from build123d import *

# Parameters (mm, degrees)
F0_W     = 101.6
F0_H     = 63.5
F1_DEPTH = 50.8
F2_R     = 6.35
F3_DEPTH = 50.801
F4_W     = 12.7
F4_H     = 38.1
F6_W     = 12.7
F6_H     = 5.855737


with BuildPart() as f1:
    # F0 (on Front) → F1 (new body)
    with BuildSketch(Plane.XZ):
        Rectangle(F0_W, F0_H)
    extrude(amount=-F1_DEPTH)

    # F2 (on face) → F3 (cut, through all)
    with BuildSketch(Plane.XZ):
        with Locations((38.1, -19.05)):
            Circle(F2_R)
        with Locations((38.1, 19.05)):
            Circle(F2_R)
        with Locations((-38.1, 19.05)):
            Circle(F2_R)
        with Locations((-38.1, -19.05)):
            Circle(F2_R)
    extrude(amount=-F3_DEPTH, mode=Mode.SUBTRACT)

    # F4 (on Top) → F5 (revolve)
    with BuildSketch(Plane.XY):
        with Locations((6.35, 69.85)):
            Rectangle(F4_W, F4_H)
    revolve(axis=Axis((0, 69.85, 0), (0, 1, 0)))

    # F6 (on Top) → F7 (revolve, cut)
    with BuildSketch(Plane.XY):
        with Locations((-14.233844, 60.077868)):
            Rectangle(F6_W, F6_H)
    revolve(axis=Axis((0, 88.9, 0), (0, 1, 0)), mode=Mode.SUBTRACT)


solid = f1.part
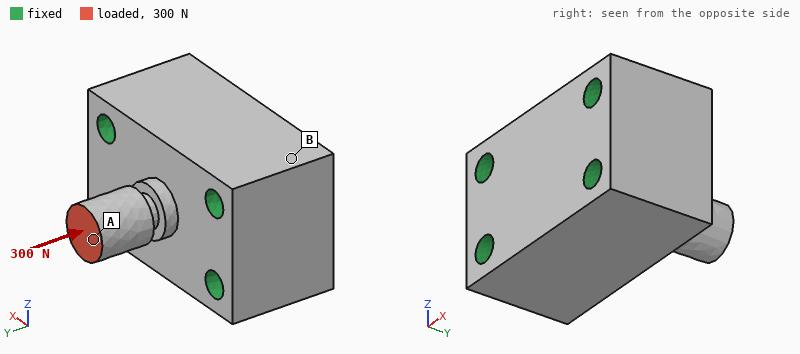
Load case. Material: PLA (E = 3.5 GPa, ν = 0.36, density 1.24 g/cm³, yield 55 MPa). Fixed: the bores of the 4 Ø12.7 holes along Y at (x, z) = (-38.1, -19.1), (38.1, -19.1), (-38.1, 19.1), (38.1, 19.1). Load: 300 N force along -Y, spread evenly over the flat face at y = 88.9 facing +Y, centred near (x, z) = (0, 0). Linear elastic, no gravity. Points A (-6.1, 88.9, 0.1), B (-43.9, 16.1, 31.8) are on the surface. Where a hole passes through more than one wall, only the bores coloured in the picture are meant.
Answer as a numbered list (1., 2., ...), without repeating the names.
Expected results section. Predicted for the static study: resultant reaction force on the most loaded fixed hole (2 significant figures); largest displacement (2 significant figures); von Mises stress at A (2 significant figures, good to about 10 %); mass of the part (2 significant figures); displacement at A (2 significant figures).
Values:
1. 80 N
2. 13 µm
3. 0.59 MPa
4. 400 g
5. 13 µm
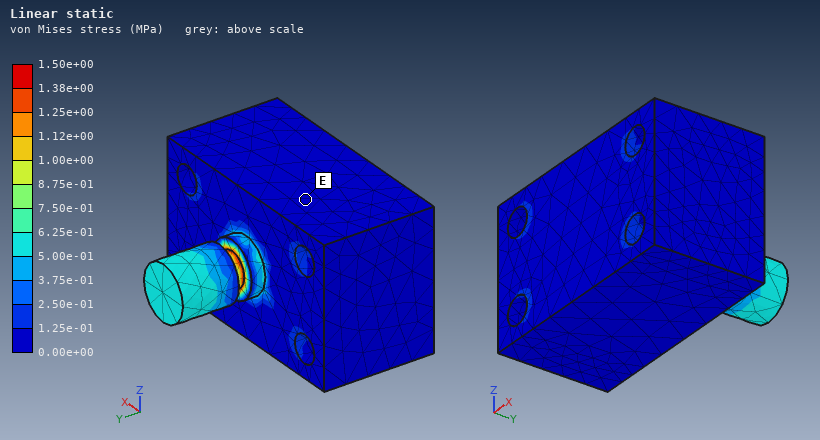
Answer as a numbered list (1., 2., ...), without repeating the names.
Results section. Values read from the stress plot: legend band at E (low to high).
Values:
1. 0.00e+00 to 1.25e-01 MPa
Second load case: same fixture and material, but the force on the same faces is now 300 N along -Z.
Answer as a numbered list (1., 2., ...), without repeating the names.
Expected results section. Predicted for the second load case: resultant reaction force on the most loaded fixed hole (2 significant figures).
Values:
1. 190 N
